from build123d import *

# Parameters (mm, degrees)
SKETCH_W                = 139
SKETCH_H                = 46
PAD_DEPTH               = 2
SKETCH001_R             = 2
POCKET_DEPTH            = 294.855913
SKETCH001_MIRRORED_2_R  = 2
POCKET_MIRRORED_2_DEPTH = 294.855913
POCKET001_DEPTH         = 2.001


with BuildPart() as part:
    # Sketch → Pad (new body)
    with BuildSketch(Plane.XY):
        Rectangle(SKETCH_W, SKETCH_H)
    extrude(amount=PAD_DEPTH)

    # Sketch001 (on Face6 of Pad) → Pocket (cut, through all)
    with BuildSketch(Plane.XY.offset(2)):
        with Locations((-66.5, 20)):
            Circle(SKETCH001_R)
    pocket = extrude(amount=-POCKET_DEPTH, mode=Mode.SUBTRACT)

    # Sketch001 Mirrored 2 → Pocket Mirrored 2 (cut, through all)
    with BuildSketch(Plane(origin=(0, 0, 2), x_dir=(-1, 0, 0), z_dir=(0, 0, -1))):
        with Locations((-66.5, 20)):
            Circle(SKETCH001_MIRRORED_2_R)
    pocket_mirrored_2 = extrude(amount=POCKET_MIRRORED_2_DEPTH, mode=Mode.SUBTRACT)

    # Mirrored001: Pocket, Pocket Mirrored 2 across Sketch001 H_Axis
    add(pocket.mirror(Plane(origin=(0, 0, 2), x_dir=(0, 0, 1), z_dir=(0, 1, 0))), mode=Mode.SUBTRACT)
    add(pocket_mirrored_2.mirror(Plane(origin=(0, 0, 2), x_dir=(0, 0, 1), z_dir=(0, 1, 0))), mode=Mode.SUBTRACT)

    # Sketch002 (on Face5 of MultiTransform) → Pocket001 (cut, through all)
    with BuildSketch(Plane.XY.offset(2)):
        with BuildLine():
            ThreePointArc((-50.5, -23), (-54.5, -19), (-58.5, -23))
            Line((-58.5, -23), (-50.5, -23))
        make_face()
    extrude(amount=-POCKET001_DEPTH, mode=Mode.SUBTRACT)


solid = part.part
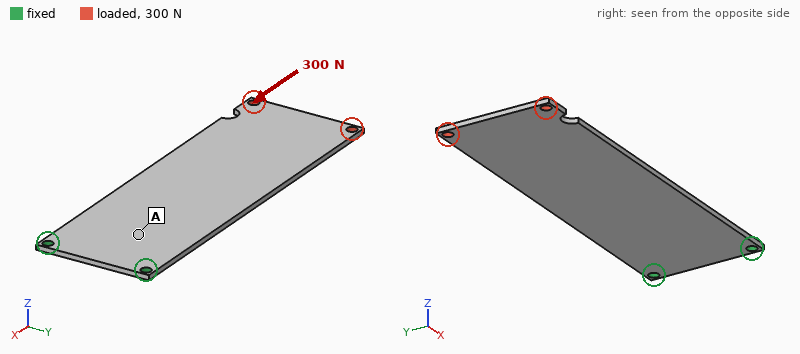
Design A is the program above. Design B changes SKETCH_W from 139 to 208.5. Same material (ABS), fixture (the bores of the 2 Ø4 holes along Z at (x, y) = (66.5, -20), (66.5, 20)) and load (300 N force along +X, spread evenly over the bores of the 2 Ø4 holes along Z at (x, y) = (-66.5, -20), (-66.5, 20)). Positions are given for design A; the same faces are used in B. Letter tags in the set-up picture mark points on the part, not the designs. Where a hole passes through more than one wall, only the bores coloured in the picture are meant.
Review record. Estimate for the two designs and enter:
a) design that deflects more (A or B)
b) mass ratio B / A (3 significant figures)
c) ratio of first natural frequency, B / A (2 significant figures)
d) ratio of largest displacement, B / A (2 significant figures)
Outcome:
A
1.51
0.65
0.67
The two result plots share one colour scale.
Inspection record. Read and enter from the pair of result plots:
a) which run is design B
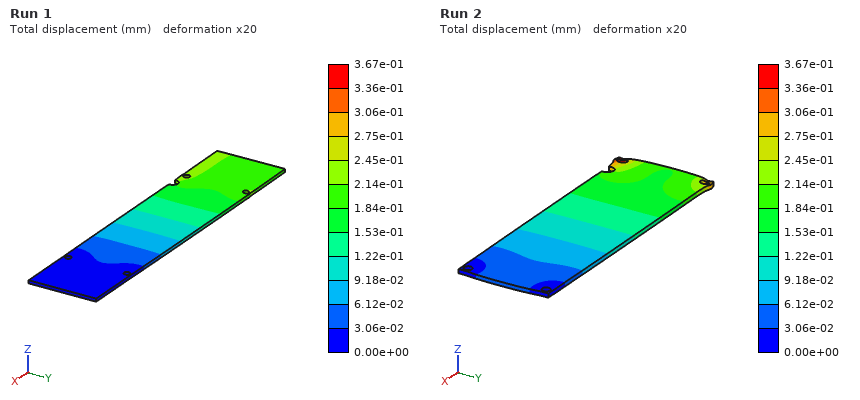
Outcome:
Run 1
